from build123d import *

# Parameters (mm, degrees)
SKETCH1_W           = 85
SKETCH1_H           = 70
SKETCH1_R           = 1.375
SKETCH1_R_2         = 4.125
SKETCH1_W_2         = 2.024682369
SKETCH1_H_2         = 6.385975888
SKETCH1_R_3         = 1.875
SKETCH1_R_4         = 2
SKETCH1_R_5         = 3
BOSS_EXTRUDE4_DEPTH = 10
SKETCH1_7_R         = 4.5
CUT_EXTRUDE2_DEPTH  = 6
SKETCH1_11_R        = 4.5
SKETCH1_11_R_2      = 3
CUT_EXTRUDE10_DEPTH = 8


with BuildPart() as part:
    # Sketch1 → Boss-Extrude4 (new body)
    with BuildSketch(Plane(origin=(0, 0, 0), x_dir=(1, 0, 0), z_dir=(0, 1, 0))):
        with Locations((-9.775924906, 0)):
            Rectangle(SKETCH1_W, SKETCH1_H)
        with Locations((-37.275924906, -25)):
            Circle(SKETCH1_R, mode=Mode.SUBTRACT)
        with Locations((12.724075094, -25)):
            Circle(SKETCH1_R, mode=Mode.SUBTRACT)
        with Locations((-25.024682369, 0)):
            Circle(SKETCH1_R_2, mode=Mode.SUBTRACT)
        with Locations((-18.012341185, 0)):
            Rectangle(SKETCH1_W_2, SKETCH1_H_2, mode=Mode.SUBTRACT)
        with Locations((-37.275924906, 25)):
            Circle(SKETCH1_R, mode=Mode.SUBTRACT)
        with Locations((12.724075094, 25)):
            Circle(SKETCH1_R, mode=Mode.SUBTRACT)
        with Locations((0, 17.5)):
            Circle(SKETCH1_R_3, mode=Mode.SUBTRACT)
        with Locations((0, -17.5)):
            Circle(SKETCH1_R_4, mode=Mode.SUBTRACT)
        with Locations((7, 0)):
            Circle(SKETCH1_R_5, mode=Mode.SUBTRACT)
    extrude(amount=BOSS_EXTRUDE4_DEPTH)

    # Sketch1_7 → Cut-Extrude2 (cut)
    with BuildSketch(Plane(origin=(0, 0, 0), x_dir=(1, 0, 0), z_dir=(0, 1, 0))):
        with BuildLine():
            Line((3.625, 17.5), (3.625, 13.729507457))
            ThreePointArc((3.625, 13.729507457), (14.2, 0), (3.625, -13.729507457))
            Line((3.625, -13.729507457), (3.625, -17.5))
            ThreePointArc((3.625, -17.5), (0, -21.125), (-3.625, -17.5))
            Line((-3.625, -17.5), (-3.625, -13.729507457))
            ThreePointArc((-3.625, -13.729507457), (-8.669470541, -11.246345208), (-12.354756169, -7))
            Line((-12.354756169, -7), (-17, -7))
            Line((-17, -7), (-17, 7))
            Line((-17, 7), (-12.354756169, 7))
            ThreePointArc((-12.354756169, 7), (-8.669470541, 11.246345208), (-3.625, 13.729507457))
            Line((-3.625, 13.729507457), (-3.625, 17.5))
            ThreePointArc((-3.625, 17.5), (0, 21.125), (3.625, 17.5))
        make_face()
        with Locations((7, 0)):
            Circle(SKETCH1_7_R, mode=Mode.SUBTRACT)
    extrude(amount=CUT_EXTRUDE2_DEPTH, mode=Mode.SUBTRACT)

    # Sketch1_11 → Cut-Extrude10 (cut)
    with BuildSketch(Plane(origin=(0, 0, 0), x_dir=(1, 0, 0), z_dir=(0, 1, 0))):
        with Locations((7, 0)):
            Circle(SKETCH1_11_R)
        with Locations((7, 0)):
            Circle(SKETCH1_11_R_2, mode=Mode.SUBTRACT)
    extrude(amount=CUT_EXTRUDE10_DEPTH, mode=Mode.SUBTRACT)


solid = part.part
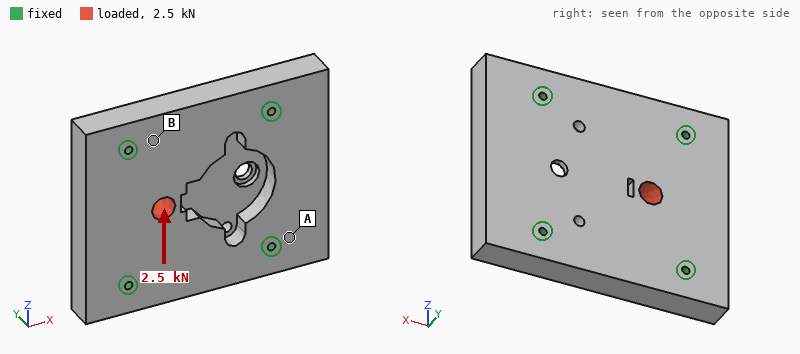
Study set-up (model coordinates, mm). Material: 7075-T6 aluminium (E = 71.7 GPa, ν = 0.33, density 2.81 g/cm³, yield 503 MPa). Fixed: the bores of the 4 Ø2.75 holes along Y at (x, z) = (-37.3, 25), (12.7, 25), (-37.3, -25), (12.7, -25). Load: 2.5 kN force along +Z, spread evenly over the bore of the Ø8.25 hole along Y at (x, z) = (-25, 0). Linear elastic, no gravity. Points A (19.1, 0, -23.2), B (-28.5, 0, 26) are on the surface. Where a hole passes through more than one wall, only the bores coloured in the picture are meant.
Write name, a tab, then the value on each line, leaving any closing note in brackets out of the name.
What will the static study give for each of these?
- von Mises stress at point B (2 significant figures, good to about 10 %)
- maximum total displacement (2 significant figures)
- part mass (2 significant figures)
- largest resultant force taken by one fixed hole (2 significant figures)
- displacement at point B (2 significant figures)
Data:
von Mises stress at point B	3.3 MPa
maximum total displacement	3.3 µm
part mass	150 g
largest resultant force taken by one fixed hole	1.0 kN
displacement at point B	1.2 µm
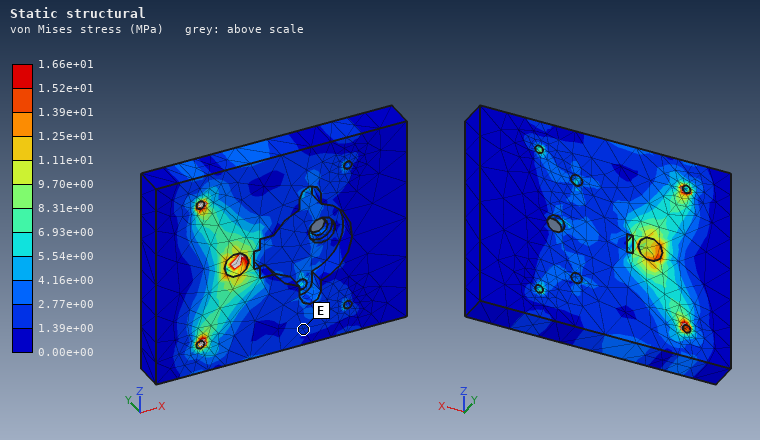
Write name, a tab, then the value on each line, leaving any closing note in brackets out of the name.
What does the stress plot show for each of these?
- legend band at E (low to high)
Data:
legend band at E	1.39e+00 to 2.77e+00 MPa
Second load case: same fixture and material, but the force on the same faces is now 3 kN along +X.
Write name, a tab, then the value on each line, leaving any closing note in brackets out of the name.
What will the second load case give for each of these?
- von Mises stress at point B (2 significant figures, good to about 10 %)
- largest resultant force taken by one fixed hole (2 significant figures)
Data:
von Mises stress at point B	3.4 MPa
largest resultant force taken by one fixed hole	1.0 kN
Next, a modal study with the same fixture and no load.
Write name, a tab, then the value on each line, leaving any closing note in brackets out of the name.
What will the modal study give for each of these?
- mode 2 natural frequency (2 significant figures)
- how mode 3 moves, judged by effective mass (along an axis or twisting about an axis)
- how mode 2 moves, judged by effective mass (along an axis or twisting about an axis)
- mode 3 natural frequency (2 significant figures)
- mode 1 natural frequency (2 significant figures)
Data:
mode 2 natural frequency	11 kHz
how mode 3 moves, judged by effective mass	twisting about Z
how mode 2 moves, judged by effective mass	along Y
mode 3 natural frequency	13 kHz
mode 1 natural frequency	9800 Hz
